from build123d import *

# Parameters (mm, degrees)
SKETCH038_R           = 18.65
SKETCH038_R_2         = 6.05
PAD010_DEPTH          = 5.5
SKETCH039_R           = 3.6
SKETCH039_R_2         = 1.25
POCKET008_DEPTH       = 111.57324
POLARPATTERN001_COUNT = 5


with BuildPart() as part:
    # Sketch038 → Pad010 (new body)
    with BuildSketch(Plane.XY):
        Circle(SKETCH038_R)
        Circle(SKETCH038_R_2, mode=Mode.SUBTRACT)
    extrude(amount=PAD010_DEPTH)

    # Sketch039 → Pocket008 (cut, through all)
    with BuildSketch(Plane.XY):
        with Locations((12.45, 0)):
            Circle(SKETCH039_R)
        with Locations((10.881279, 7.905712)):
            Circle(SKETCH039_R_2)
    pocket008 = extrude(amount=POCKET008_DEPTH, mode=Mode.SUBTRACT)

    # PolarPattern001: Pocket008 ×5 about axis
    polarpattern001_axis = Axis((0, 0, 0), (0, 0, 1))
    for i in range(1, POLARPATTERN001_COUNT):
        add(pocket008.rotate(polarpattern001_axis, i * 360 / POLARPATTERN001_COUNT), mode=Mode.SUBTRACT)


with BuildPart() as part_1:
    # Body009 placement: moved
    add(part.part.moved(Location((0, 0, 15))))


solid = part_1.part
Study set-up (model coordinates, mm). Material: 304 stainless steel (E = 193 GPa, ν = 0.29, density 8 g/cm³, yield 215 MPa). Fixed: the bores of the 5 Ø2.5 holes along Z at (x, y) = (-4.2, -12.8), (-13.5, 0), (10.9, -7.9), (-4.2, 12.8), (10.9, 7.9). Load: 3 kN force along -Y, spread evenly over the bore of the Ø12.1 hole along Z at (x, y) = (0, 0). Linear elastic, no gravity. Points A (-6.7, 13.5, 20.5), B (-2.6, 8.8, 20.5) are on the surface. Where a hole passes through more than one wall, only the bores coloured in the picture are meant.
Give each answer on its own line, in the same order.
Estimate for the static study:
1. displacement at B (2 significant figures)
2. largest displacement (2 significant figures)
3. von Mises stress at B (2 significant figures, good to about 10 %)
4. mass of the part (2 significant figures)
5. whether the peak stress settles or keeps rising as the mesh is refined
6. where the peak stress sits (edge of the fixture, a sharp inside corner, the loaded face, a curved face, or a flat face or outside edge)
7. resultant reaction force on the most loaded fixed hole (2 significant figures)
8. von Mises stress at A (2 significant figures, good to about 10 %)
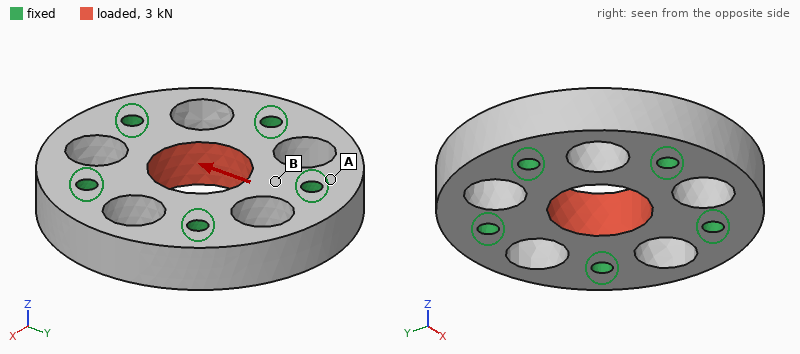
0.45 µm
1.3 µm
18 MPa
33 g
keeps rising
edge of the fixture
850 N
7.1 MPa
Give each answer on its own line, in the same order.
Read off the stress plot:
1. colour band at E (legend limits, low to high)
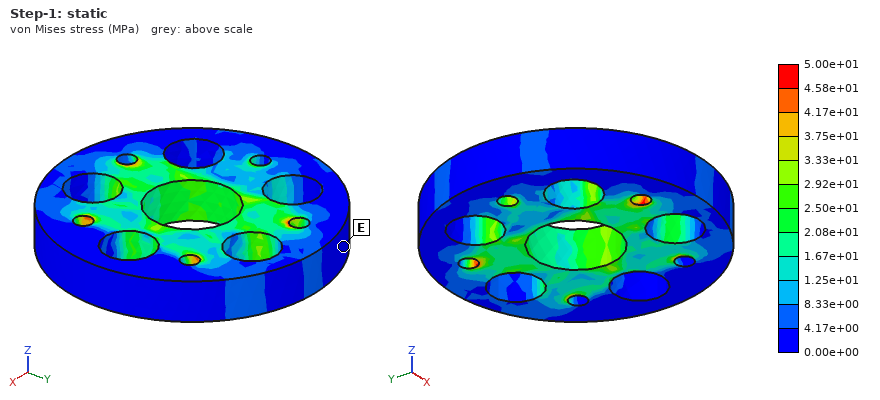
0.00e+00 to 4.17e+00 MPa
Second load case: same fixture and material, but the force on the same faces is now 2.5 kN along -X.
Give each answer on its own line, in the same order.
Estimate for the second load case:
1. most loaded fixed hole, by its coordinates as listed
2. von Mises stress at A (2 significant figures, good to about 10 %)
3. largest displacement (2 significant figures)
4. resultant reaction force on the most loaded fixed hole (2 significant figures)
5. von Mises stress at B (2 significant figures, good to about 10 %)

(-13.5, 0)
7.3 MPa
1.1 µm
740 N
9.4 MPa
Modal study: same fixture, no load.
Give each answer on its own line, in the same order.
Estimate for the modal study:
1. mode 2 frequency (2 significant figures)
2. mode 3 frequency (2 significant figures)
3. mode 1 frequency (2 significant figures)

50 kHz
53 kHz
50 kHz
